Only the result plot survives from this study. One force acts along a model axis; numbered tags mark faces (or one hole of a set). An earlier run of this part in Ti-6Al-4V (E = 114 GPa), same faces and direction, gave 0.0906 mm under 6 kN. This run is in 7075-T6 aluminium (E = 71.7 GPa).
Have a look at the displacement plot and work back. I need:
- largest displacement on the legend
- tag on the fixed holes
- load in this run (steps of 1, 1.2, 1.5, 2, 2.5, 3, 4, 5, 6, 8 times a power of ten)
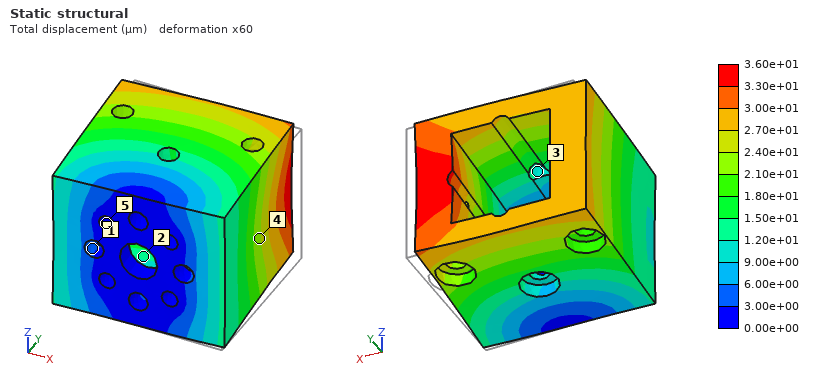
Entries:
3.60e+01 µm
5
1.5 kN
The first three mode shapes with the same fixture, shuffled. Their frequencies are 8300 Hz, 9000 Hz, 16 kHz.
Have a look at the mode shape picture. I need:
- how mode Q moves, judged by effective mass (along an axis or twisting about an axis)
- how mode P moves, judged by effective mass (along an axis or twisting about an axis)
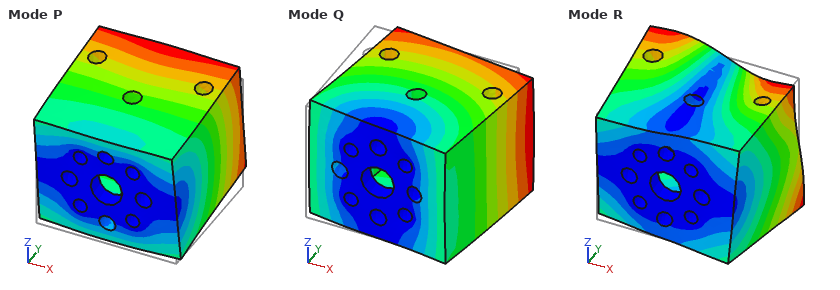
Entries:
along X
along Z
